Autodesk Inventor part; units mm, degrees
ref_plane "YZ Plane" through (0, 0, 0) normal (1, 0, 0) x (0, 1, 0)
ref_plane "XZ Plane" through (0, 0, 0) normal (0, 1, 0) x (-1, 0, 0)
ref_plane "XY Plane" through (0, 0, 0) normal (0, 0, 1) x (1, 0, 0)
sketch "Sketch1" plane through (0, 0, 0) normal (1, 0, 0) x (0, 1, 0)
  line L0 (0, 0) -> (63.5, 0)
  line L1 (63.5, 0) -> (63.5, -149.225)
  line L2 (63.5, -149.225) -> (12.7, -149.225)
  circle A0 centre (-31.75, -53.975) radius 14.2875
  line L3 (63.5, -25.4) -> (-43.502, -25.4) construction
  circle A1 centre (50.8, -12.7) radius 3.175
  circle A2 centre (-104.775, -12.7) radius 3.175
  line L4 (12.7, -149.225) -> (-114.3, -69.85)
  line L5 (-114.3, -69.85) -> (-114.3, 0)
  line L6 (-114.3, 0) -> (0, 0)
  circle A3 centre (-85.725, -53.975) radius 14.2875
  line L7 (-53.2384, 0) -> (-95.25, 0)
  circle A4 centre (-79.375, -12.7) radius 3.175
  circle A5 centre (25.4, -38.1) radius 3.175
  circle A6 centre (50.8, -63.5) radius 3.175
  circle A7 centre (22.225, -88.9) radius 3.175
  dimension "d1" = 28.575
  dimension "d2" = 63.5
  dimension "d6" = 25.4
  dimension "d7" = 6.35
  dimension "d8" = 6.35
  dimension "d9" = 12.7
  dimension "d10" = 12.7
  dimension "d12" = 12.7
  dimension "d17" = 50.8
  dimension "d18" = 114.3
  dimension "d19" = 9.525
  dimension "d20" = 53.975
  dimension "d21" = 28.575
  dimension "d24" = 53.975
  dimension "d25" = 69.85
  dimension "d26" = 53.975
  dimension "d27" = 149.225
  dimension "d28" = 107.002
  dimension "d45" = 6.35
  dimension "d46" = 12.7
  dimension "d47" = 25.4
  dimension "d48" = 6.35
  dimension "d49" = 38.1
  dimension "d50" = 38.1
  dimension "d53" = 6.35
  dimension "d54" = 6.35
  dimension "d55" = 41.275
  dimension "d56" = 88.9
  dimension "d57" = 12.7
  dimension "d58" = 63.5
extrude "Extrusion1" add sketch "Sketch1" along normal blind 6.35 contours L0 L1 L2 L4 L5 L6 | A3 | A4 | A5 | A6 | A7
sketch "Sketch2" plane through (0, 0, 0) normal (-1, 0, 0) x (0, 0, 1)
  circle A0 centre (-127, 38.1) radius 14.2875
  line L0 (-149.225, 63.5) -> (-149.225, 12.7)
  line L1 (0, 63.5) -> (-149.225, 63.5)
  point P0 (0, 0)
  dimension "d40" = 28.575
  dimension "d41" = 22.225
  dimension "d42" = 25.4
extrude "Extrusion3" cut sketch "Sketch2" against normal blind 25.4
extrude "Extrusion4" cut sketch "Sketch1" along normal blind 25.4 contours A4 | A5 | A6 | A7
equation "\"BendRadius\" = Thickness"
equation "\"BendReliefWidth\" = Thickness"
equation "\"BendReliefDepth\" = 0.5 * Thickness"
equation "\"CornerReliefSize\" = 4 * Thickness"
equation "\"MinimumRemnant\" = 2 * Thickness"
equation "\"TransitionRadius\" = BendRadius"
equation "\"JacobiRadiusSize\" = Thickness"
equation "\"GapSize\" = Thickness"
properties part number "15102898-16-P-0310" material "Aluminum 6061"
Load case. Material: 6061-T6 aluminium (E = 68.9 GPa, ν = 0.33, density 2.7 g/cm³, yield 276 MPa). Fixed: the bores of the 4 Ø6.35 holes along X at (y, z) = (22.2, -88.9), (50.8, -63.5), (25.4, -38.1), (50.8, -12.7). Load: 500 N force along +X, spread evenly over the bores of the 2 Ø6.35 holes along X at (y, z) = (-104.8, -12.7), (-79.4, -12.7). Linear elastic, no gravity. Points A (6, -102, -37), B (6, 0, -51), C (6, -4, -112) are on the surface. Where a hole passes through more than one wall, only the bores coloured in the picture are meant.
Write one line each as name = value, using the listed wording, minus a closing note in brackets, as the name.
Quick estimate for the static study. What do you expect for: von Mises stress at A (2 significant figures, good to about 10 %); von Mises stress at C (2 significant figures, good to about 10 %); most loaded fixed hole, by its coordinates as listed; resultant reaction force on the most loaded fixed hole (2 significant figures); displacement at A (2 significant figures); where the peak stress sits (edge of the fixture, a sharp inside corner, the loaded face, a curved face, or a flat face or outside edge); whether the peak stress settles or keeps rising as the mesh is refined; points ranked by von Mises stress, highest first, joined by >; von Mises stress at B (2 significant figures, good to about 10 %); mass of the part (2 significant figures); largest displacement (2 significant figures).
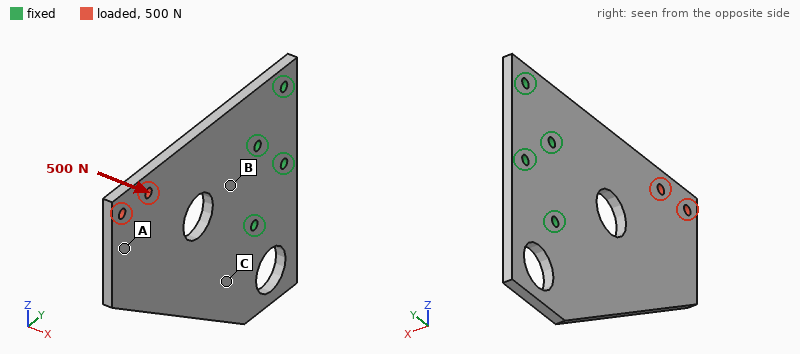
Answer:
von Mises stress at A = 18 MPa
von Mises stress at C = 36 MPa
most loaded fixed hole, by its coordinates as listed = (25.4, -38.1)
resultant reaction force on the most loaded fixed hole = 1.2 kN
displacement at A = 2.1 mm
where the peak stress sits = edge of the fixture
whether the peak stress settles or keeps rising as the mesh is refined = keeps rising
points ranked by von Mises stress, highest first, joined by > = B > C > A
von Mises stress at B = 54 MPa
mass of the part = 340 g
largest displacement = 2.8 mm
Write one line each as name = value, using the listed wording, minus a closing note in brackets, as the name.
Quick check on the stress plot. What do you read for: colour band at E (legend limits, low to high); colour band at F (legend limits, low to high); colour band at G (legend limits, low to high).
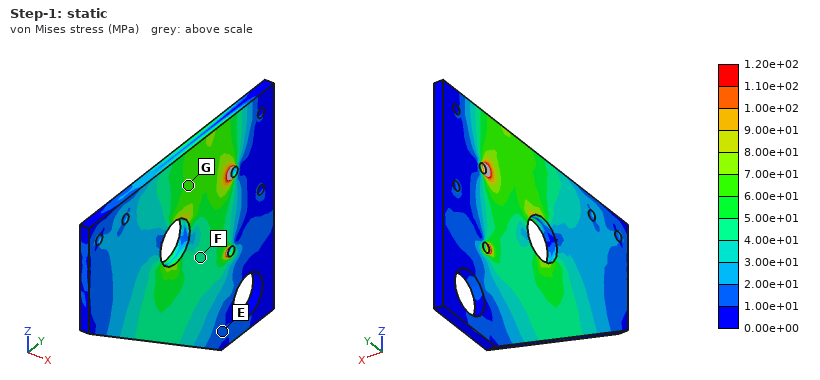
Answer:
colour band at E = 1.00e+01 to 2.00e+01 MPa
colour band at F = 4.00e+01 to 5.00e+01 MPa
colour band at G = 6.00e+01 to 7.00e+01 MPa
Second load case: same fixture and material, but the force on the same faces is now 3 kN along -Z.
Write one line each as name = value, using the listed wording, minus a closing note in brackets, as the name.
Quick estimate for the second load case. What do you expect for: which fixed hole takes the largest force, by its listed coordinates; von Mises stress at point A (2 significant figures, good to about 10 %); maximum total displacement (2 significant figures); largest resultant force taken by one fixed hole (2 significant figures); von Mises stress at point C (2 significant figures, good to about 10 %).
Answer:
which fixed hole takes the largest force, by its listed coordinates = (22.2, -88.9)
von Mises stress at point A = 9.0 MPa
maximum total displacement = 95 µm
largest resultant force taken by one fixed hole = 5.1 kN
von Mises stress at point C = 9.0 MPa
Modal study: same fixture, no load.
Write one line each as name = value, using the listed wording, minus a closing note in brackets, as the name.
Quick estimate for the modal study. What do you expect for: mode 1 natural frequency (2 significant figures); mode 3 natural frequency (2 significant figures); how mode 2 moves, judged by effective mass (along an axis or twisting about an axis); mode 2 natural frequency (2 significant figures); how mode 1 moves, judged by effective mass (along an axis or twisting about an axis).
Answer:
mode 1 natural frequency = 310 Hz
mode 3 natural frequency = 1500 Hz
how mode 2 moves, judged by effective mass = twisting about Y
mode 2 natural frequency = 920 Hz
how mode 1 moves, judged by effective mass = along X
